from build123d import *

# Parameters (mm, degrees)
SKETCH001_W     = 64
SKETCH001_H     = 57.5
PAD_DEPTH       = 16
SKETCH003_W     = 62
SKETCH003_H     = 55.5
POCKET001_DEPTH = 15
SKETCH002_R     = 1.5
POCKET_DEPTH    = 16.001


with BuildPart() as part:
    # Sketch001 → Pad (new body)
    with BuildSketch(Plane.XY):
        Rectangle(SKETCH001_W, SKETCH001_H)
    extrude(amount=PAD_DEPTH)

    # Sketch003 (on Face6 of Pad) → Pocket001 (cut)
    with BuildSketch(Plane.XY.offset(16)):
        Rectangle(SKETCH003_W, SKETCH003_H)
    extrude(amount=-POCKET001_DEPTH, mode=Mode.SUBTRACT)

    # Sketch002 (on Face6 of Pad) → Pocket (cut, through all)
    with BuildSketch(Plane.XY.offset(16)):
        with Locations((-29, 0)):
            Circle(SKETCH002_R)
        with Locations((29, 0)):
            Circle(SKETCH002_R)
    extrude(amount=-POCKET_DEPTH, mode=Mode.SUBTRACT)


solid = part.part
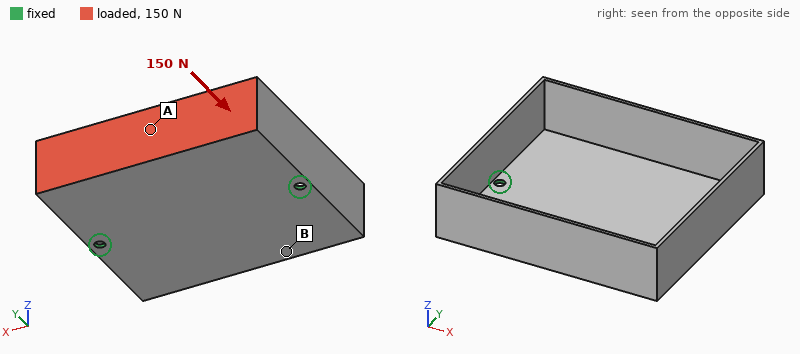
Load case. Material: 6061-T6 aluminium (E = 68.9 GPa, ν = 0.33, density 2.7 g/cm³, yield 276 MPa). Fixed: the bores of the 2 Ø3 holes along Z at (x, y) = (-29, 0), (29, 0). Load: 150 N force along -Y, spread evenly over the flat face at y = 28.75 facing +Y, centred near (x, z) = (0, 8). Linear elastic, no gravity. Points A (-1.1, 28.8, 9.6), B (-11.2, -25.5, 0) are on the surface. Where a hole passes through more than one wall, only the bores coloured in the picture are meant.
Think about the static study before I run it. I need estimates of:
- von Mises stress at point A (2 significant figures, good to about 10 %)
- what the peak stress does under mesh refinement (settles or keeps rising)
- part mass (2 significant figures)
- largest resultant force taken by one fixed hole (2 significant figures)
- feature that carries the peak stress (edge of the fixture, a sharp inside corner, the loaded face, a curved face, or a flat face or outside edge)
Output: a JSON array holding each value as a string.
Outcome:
["14 MPa", "keeps rising", "20 g", "76 N", "edge of the fixture"]
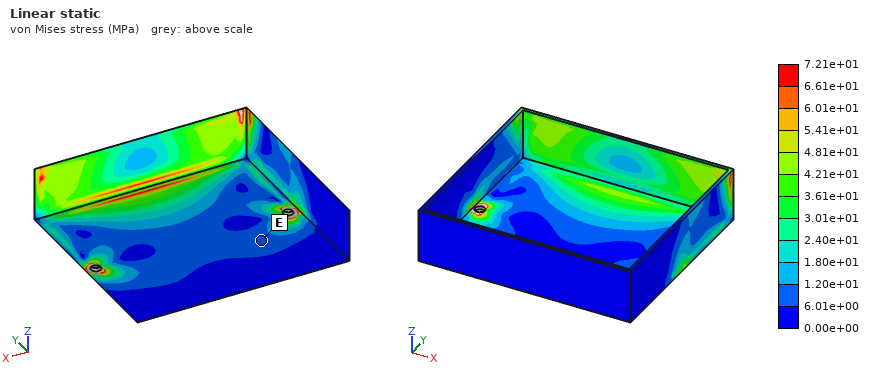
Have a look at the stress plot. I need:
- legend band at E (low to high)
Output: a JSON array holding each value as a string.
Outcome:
["6.01e+00 to 1.20e+01 MPa"]
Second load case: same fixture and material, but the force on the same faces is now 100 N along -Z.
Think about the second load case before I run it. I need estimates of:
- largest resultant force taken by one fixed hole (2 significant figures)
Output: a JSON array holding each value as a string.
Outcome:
["52 N"]
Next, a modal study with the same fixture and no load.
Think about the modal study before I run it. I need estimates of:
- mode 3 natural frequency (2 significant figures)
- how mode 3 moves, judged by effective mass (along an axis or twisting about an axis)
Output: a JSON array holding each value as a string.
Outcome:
["2000 Hz", "along Z"]
